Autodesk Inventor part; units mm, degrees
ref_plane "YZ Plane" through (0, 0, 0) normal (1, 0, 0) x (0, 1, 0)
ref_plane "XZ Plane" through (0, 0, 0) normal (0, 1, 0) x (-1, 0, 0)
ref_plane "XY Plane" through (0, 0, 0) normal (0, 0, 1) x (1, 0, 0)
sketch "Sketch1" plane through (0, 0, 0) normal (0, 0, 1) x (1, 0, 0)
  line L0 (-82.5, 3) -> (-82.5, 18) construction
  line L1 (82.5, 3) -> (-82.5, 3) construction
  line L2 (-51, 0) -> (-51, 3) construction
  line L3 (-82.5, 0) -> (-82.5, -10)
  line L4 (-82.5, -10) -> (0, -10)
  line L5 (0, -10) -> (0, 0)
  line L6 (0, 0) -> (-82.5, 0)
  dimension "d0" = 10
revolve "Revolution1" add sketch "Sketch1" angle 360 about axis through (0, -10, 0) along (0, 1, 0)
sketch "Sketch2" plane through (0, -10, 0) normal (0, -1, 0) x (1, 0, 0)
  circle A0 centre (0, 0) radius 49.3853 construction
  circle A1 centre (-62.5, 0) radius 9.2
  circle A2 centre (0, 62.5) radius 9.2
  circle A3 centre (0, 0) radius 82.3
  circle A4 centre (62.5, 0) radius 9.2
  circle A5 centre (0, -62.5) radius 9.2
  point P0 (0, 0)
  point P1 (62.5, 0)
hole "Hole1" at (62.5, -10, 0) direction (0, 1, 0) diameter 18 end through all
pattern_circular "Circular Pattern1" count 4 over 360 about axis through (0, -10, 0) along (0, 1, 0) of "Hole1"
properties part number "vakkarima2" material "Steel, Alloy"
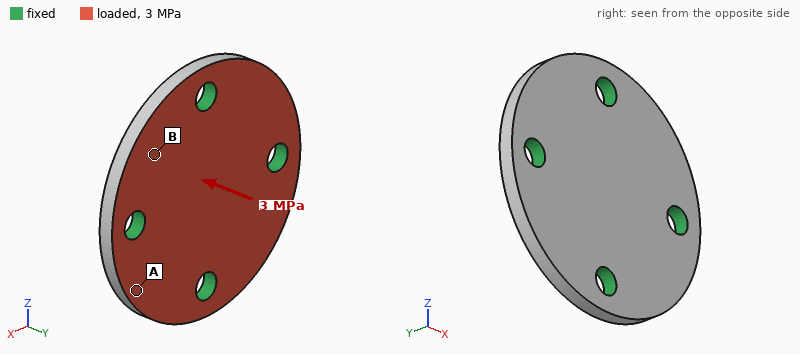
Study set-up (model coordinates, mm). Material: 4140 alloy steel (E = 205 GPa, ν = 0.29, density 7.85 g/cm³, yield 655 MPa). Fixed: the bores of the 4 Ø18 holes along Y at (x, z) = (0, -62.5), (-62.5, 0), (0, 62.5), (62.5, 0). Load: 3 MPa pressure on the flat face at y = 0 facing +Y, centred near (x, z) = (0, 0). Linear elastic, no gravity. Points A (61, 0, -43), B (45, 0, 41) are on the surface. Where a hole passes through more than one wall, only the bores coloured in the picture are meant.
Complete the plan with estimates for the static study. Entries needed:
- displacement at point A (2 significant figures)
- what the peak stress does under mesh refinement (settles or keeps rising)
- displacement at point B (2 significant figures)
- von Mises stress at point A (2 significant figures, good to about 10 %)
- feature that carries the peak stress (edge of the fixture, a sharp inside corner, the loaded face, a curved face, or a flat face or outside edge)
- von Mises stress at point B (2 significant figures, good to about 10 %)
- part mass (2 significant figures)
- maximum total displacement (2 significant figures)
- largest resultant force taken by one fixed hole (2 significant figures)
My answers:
37 µm
keeps rising
31 µm
38 MPa
edge of the fixture
55 MPa
1.6 kg
48 µm
15 kN
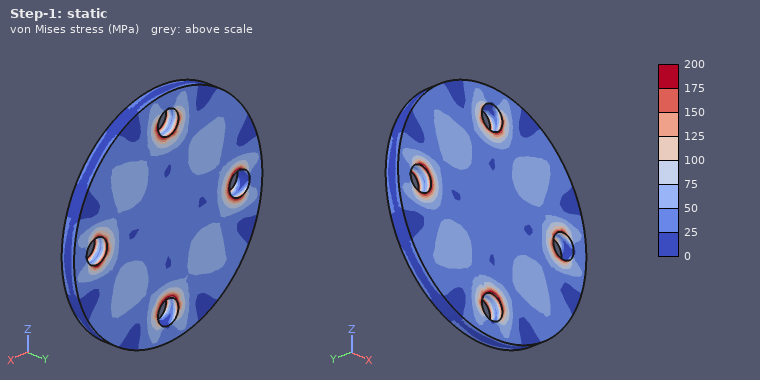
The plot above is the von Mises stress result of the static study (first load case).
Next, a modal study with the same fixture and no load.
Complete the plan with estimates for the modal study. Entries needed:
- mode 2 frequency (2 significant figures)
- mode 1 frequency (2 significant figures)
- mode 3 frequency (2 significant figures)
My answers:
5600 Hz
5500 Hz
5600 Hz
